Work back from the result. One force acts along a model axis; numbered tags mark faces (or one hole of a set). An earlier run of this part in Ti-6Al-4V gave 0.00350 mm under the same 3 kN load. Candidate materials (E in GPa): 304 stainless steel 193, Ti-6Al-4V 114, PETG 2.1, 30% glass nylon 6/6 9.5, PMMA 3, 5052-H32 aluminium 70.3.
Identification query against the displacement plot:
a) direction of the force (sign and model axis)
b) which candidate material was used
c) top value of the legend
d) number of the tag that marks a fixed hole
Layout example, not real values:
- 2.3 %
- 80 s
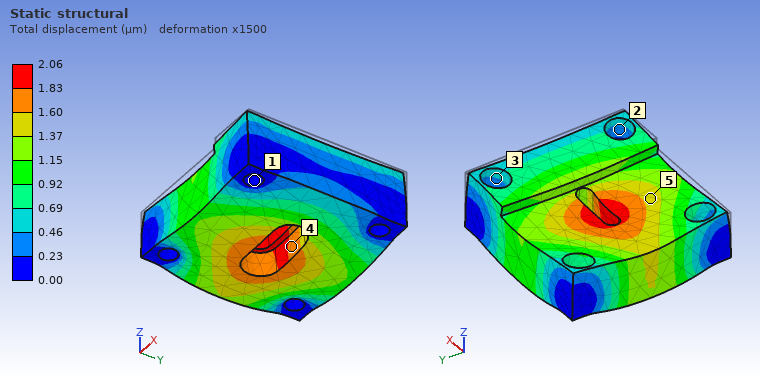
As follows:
- -Z
- 304 stainless steel
- 2.06 µm
- 1
